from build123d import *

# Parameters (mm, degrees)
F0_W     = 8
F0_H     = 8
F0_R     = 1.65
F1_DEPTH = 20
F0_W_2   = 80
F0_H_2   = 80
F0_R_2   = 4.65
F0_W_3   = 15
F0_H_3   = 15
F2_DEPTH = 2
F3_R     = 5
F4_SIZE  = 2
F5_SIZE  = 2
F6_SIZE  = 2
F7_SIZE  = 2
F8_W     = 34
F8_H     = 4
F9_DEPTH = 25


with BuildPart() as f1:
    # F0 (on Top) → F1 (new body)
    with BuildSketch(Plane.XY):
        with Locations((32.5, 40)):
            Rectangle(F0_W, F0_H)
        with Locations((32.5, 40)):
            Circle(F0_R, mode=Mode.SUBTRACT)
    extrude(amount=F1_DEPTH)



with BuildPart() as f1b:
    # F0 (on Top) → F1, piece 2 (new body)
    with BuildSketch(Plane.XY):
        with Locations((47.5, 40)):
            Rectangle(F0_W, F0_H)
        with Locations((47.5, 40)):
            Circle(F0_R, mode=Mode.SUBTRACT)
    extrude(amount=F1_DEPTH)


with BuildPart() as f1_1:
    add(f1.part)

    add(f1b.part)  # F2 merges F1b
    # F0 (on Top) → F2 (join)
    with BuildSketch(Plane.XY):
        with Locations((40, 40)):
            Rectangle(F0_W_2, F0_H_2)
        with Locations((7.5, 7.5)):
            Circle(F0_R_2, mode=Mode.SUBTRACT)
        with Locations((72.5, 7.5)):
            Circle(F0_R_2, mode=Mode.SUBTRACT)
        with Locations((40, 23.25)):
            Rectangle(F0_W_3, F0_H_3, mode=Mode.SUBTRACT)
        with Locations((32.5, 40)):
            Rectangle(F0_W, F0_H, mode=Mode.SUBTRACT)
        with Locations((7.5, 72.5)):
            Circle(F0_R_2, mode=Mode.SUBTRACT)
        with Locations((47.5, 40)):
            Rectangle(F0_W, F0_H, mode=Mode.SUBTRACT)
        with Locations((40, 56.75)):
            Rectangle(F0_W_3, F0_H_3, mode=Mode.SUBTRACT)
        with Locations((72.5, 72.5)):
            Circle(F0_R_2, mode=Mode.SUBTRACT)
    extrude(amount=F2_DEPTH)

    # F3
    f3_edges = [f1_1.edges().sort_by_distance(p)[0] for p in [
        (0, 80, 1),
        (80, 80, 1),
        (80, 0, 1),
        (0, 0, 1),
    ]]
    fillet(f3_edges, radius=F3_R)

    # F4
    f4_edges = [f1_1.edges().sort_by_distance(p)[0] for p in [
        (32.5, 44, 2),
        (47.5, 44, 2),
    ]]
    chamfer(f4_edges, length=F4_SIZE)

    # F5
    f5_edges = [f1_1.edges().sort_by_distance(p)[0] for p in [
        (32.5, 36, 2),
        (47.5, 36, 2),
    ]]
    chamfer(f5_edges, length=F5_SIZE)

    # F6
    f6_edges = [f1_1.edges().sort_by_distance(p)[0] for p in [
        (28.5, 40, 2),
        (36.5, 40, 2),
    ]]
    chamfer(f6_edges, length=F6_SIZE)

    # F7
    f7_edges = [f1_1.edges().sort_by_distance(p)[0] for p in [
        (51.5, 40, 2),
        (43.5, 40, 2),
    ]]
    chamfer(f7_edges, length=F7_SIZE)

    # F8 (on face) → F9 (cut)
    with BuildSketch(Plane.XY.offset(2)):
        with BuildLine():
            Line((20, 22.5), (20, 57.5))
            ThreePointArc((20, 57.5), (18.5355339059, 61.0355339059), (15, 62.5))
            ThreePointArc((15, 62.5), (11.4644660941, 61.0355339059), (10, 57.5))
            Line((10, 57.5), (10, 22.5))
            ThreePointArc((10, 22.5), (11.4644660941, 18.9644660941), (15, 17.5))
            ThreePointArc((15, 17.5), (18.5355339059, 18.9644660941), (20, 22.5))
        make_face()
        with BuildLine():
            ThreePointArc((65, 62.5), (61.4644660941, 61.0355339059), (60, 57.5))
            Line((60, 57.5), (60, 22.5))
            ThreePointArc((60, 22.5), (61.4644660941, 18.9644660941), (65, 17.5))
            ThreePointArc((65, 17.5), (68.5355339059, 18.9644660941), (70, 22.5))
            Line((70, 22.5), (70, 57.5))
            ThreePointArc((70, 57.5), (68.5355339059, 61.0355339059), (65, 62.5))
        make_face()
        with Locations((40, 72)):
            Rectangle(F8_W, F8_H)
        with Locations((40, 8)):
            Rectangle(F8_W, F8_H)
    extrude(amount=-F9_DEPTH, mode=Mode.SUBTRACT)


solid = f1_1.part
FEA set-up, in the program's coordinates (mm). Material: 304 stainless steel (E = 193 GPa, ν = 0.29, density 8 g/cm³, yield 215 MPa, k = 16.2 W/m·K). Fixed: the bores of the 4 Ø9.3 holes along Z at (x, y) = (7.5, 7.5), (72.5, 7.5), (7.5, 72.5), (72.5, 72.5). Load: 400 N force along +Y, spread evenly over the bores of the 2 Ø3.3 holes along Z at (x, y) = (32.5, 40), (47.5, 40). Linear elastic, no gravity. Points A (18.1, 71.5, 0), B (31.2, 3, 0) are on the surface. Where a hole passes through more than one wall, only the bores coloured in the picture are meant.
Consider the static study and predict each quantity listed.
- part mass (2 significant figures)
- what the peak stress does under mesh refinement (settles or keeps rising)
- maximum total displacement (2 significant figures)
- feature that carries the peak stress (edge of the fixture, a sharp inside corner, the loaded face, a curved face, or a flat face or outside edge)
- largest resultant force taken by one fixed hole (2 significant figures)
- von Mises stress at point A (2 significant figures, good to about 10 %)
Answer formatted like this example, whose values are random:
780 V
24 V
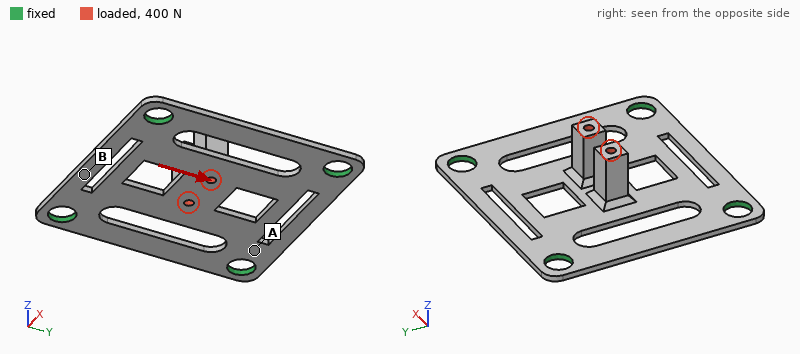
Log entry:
89 g
keeps rising
66 µm
a sharp inside corner
120 N
28 MPa
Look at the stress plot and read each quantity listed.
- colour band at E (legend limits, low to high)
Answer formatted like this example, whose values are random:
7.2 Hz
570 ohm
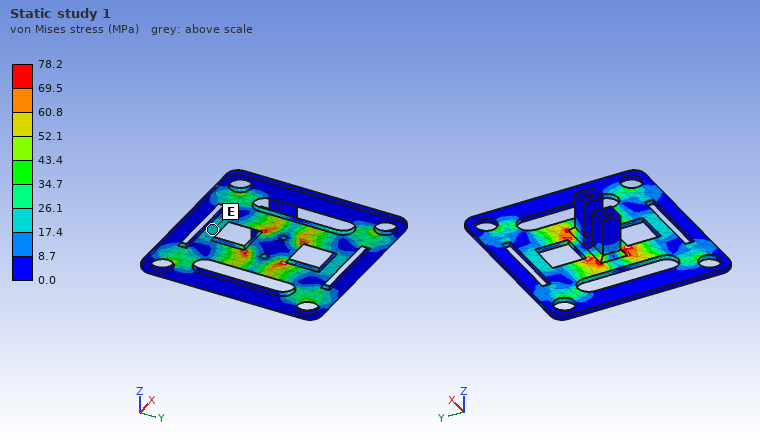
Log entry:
17.4 to 26.1 MPa
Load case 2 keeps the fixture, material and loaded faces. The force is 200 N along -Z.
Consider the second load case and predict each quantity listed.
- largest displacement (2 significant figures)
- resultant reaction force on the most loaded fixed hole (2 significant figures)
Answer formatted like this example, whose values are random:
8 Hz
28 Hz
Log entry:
91 µm
54 N
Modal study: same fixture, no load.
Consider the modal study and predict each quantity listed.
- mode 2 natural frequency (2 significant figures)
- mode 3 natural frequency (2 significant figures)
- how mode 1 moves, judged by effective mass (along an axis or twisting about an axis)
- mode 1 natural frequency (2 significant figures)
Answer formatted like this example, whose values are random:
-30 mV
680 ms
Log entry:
2400 Hz
2700 Hz
along Z
1300 Hz
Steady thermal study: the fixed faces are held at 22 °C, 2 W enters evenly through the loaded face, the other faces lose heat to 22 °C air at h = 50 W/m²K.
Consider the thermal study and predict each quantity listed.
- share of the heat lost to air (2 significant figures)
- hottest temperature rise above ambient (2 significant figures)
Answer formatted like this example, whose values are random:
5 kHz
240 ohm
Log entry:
91 %
14 K
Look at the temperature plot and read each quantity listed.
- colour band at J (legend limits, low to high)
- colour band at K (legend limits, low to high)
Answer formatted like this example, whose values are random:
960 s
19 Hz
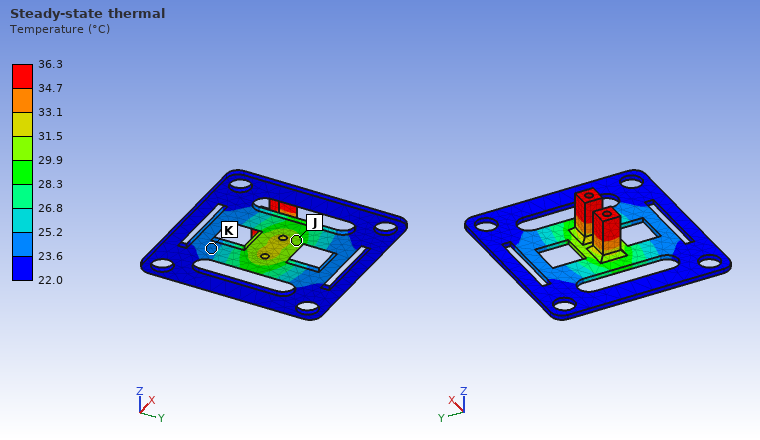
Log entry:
29.9 to 31.5 °C
23.6 to 25.2 °C
